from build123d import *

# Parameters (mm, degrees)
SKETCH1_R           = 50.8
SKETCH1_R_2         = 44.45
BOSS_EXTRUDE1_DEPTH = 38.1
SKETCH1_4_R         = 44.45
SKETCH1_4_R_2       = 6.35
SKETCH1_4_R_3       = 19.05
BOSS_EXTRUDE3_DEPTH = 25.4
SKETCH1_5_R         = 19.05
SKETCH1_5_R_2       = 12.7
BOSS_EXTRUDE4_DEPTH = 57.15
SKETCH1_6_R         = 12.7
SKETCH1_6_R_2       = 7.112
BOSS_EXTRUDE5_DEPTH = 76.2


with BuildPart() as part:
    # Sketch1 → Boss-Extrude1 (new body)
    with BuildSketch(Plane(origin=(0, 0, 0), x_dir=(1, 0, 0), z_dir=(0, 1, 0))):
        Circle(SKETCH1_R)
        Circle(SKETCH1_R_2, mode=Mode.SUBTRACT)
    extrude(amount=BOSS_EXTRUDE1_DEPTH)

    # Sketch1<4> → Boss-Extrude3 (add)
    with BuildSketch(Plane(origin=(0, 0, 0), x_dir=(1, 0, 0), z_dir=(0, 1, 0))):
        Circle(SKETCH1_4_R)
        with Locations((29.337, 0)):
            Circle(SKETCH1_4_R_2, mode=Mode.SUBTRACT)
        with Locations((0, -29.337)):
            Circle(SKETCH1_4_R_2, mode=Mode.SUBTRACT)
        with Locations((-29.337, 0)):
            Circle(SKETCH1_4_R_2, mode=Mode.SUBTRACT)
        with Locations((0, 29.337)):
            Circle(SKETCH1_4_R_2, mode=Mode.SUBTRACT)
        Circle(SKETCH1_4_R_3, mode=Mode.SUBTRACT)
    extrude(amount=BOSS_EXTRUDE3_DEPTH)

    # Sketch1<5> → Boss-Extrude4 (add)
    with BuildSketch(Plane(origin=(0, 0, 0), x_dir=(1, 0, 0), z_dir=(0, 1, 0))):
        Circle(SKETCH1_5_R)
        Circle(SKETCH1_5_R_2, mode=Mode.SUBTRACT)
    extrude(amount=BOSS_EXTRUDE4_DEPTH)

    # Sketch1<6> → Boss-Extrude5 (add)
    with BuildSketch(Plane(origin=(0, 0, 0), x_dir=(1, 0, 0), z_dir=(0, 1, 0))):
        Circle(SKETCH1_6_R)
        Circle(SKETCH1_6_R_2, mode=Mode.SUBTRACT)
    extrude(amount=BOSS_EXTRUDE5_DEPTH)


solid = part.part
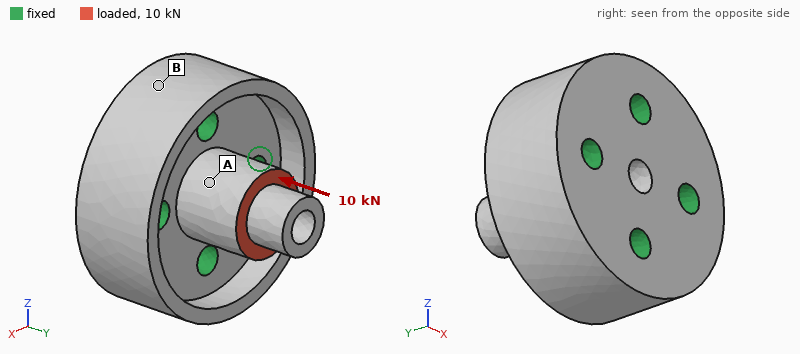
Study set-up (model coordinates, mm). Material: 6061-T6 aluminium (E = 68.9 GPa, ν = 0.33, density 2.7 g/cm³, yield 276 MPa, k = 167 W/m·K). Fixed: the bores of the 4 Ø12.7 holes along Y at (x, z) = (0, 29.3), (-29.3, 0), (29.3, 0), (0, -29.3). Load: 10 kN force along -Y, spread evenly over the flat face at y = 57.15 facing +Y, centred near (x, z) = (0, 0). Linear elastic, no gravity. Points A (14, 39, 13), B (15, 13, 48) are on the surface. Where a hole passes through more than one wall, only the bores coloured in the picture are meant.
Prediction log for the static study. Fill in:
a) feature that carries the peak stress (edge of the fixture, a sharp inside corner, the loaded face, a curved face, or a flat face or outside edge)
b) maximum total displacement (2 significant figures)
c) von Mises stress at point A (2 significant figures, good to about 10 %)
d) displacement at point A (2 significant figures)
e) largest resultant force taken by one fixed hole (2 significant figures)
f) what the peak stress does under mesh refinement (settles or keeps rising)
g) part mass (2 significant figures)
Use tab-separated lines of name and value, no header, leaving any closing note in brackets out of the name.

feature that carries the peak stress	edge of the fixture
maximum total displacement	7.8 µm
von Mises stress at point A	9.9 MPa
displacement at point A	4.2 µm
largest resultant force taken by one fixed hole	2.7 kN
what the peak stress does under mesh refinement	keeps rising
part mass	680 g
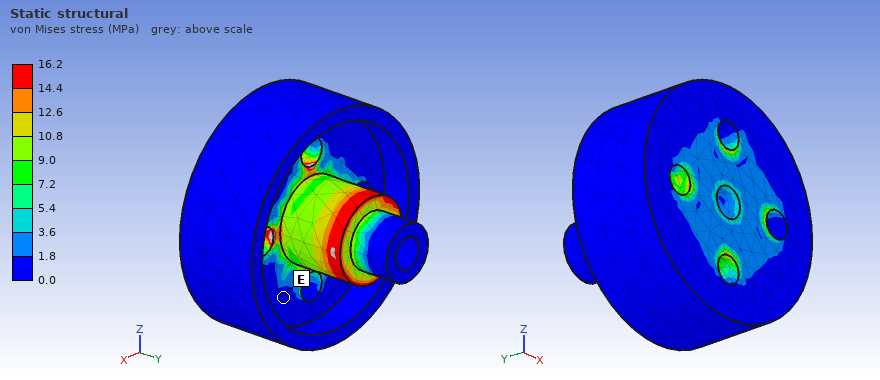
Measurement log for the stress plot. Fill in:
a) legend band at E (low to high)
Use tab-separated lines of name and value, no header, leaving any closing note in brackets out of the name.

legend band at E	0.0 to 1.8 MPa
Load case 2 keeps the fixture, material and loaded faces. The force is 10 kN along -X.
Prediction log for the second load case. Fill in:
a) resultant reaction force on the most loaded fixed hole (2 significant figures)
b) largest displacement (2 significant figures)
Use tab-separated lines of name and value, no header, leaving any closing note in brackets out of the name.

resultant reaction force on the most loaded fixed hole	8.2 kN
largest displacement	65 µm
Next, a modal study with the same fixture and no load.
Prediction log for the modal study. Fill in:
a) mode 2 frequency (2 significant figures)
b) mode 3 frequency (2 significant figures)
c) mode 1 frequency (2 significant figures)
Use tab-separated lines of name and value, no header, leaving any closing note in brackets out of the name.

mode 2 frequency	9300 Hz
mode 3 frequency	15 kHz
mode 1 frequency	9300 Hz
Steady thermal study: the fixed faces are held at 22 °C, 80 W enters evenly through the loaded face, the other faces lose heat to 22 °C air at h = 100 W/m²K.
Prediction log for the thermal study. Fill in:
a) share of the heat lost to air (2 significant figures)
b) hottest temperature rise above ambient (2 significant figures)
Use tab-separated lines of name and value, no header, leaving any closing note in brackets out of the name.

share of the heat lost to air	13 %
hottest temperature rise above ambient	19 K
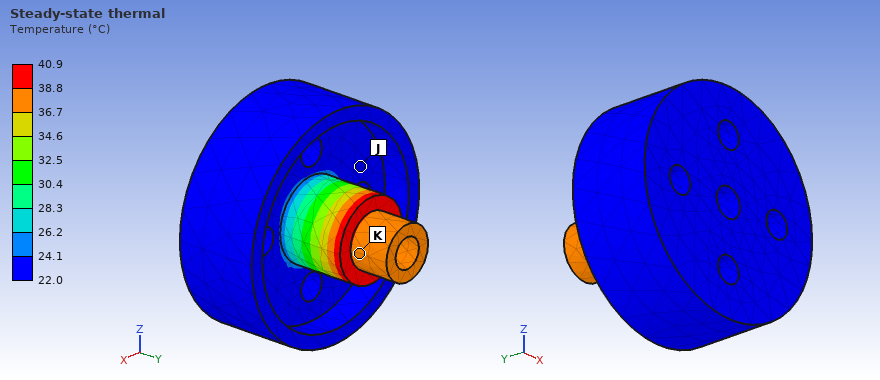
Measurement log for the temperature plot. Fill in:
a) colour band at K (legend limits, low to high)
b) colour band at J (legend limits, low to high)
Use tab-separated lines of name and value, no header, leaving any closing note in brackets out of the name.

colour band at K	36.7 to 38.8 °C
colour band at J	22.0 to 24.1 °C
